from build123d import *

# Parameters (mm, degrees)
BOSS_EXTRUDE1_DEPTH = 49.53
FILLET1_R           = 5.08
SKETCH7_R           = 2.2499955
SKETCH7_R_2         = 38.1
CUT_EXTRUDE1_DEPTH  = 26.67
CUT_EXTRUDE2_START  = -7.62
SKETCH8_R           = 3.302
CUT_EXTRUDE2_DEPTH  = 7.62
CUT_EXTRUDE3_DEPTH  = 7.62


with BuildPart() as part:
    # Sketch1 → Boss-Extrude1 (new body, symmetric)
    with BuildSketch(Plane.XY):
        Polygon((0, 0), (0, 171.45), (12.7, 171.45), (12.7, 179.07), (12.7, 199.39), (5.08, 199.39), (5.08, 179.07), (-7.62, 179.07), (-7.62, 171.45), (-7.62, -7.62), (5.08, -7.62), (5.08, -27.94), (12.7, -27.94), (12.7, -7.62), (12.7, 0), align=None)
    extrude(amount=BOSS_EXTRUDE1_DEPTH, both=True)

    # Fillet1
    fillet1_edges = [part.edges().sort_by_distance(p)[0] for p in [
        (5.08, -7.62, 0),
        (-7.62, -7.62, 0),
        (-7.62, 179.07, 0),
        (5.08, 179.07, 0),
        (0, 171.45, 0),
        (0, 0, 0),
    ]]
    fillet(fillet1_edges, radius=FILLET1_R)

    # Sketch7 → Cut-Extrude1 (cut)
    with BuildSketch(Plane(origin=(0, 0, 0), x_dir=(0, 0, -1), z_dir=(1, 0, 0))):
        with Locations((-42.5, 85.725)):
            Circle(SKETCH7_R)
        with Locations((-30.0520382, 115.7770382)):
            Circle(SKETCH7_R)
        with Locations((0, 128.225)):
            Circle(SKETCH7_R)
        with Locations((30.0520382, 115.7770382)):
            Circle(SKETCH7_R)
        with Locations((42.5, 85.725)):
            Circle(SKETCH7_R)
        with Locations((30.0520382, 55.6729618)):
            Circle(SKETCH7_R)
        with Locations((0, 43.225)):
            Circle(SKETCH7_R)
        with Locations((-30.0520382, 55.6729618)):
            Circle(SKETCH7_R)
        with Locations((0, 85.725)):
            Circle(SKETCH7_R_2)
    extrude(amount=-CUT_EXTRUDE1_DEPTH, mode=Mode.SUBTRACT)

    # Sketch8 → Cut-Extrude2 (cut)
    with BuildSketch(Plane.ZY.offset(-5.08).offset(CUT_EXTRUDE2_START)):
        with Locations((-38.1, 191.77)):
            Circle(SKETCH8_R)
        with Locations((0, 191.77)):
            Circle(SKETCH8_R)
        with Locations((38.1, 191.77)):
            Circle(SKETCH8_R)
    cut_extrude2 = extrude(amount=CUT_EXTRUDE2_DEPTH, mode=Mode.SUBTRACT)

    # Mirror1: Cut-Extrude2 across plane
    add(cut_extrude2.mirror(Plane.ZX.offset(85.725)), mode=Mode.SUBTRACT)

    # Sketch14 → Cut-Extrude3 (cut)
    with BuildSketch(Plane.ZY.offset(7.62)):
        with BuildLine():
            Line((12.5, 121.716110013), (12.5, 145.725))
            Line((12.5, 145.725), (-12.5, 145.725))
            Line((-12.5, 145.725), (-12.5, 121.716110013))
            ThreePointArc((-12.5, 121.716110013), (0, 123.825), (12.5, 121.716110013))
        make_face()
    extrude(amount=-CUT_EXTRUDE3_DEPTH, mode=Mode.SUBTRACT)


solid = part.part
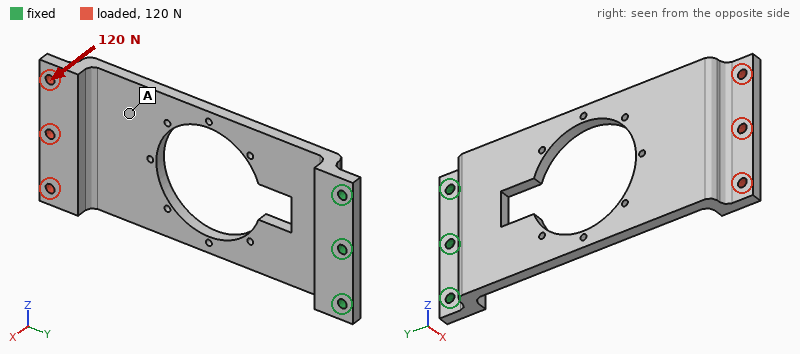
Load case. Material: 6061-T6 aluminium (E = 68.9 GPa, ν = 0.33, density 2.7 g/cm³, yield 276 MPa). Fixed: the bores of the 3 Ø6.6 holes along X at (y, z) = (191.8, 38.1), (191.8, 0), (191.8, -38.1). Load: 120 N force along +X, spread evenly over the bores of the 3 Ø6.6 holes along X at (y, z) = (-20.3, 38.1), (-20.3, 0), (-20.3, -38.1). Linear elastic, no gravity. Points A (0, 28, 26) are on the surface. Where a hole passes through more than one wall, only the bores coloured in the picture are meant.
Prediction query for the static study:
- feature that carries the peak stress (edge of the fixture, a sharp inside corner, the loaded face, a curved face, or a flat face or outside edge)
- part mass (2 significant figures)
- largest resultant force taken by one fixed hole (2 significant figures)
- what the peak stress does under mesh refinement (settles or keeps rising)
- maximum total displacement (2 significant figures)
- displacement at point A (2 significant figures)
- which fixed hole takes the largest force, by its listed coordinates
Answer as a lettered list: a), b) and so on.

a) a sharp inside corner
b) 410 g
c) 130 N
d) keeps rising
e) 2.9 mm
f) 1.7 mm
g) (191.8, 0)
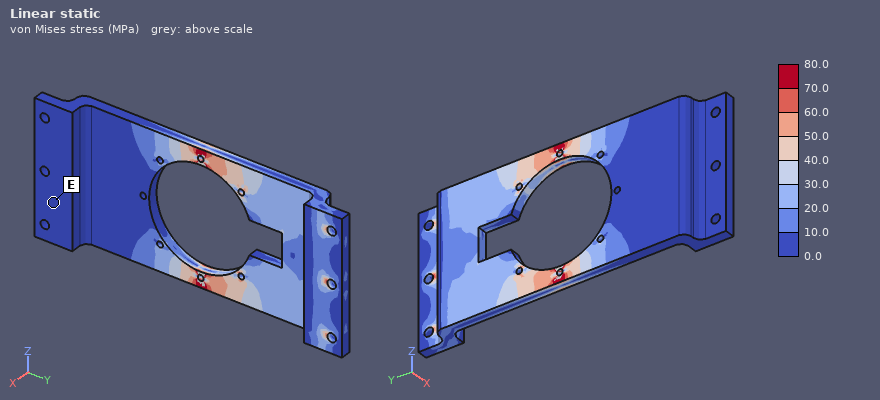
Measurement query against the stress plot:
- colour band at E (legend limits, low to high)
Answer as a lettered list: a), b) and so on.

a) 0.0 to 10.0 MPa
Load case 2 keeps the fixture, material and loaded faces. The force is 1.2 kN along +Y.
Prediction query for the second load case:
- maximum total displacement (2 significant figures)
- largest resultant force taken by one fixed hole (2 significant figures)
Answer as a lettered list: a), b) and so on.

a) 2.7 mm
b) 450 N
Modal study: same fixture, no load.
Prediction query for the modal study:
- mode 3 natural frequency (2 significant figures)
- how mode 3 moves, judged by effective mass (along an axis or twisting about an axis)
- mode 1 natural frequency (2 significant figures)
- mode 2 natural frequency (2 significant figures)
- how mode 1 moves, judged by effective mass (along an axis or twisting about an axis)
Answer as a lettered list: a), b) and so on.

a) 700 Hz
b) along Z
c) 97 Hz
d) 400 Hz
e) along X
